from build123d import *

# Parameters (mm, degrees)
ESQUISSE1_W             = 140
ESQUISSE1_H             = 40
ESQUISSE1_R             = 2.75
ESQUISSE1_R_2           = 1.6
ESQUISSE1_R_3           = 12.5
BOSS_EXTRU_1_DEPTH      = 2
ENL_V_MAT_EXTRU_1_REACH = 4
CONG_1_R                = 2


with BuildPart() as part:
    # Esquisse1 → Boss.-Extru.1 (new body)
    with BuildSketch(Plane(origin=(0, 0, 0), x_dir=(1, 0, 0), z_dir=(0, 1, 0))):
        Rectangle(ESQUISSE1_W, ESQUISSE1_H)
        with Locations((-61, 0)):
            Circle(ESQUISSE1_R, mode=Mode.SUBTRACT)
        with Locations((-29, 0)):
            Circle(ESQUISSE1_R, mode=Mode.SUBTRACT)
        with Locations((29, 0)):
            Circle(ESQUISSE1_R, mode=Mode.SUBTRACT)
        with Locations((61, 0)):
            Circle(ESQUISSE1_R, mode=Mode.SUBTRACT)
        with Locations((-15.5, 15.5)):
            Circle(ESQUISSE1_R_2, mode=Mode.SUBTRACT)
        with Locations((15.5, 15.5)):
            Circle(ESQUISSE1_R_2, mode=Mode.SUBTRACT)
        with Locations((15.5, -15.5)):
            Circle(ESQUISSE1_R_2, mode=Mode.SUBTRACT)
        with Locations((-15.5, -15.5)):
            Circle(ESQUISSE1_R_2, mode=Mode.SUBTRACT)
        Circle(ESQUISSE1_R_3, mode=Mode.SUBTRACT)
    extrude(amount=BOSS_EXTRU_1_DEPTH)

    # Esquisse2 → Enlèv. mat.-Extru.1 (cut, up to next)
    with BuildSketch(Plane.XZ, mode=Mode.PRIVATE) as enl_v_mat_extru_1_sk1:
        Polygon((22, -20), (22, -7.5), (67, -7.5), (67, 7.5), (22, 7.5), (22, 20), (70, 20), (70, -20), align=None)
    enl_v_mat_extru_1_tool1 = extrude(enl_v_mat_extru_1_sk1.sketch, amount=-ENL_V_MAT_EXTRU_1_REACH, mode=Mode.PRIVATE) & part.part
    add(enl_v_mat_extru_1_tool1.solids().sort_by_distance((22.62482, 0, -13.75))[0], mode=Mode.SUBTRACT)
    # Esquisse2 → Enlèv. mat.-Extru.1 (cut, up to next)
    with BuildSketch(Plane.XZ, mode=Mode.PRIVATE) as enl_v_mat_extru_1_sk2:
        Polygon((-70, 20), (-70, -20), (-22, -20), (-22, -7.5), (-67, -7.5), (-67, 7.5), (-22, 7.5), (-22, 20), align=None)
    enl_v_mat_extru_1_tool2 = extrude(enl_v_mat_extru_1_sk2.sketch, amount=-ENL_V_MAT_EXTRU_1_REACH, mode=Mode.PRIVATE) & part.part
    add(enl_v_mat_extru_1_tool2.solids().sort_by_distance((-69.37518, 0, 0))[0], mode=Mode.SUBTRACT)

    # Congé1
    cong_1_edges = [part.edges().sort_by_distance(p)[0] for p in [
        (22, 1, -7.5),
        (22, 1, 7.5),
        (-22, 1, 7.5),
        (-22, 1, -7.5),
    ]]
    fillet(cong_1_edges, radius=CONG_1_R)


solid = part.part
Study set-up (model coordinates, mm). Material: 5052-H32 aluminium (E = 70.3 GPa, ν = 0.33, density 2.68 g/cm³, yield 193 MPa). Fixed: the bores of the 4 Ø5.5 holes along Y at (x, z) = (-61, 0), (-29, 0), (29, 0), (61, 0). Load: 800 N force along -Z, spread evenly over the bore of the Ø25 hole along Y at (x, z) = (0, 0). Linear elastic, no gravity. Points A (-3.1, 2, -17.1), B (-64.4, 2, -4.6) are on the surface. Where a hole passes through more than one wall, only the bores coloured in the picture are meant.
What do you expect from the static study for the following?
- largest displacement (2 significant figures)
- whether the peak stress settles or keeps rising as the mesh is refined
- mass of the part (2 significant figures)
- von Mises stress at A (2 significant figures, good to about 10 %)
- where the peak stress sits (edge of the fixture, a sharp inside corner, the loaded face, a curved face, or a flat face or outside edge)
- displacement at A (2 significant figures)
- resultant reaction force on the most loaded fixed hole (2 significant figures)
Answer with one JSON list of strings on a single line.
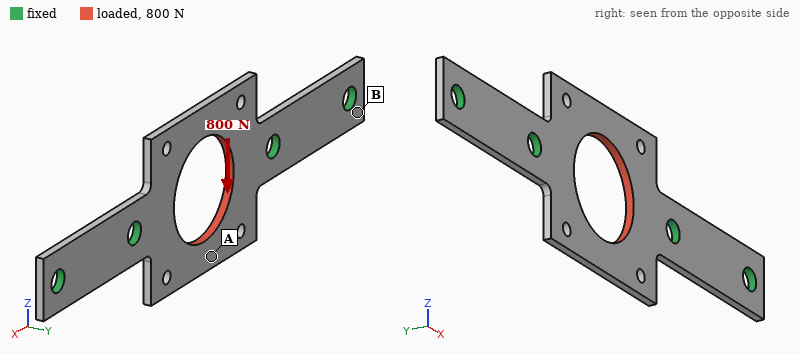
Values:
["11 µm", "keeps rising", "13 g", "14 MPa", "edge of the fixture", "10 µm", "420 N"]
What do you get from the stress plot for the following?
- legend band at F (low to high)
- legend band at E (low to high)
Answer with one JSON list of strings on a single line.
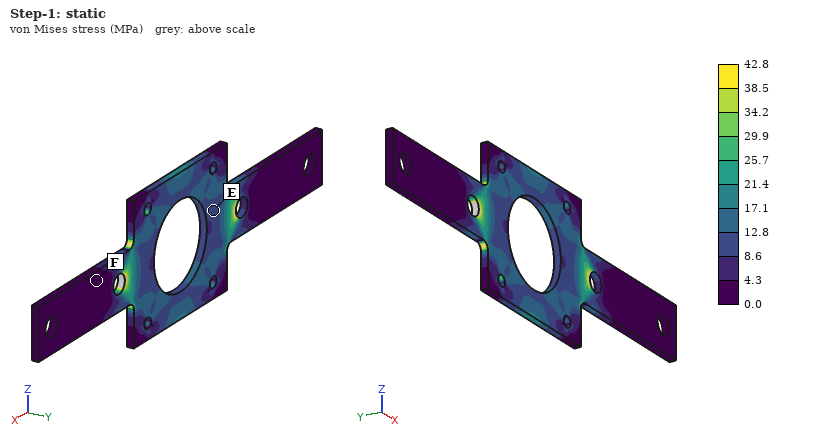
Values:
["0.0 to 4.3 MPa", "8.6 to 12.8 MPa"]
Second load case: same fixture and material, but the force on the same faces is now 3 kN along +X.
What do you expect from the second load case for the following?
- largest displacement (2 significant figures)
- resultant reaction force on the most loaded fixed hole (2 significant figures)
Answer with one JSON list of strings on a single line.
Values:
["21 µm", "1.4 kN"]
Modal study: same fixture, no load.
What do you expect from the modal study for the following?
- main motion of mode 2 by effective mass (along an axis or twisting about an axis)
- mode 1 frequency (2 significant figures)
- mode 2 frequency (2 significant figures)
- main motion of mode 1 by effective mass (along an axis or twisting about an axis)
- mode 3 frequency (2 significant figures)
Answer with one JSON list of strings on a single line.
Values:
["along Y", "2200 Hz", "2500 Hz", "twisting about X", "5100 Hz"]
